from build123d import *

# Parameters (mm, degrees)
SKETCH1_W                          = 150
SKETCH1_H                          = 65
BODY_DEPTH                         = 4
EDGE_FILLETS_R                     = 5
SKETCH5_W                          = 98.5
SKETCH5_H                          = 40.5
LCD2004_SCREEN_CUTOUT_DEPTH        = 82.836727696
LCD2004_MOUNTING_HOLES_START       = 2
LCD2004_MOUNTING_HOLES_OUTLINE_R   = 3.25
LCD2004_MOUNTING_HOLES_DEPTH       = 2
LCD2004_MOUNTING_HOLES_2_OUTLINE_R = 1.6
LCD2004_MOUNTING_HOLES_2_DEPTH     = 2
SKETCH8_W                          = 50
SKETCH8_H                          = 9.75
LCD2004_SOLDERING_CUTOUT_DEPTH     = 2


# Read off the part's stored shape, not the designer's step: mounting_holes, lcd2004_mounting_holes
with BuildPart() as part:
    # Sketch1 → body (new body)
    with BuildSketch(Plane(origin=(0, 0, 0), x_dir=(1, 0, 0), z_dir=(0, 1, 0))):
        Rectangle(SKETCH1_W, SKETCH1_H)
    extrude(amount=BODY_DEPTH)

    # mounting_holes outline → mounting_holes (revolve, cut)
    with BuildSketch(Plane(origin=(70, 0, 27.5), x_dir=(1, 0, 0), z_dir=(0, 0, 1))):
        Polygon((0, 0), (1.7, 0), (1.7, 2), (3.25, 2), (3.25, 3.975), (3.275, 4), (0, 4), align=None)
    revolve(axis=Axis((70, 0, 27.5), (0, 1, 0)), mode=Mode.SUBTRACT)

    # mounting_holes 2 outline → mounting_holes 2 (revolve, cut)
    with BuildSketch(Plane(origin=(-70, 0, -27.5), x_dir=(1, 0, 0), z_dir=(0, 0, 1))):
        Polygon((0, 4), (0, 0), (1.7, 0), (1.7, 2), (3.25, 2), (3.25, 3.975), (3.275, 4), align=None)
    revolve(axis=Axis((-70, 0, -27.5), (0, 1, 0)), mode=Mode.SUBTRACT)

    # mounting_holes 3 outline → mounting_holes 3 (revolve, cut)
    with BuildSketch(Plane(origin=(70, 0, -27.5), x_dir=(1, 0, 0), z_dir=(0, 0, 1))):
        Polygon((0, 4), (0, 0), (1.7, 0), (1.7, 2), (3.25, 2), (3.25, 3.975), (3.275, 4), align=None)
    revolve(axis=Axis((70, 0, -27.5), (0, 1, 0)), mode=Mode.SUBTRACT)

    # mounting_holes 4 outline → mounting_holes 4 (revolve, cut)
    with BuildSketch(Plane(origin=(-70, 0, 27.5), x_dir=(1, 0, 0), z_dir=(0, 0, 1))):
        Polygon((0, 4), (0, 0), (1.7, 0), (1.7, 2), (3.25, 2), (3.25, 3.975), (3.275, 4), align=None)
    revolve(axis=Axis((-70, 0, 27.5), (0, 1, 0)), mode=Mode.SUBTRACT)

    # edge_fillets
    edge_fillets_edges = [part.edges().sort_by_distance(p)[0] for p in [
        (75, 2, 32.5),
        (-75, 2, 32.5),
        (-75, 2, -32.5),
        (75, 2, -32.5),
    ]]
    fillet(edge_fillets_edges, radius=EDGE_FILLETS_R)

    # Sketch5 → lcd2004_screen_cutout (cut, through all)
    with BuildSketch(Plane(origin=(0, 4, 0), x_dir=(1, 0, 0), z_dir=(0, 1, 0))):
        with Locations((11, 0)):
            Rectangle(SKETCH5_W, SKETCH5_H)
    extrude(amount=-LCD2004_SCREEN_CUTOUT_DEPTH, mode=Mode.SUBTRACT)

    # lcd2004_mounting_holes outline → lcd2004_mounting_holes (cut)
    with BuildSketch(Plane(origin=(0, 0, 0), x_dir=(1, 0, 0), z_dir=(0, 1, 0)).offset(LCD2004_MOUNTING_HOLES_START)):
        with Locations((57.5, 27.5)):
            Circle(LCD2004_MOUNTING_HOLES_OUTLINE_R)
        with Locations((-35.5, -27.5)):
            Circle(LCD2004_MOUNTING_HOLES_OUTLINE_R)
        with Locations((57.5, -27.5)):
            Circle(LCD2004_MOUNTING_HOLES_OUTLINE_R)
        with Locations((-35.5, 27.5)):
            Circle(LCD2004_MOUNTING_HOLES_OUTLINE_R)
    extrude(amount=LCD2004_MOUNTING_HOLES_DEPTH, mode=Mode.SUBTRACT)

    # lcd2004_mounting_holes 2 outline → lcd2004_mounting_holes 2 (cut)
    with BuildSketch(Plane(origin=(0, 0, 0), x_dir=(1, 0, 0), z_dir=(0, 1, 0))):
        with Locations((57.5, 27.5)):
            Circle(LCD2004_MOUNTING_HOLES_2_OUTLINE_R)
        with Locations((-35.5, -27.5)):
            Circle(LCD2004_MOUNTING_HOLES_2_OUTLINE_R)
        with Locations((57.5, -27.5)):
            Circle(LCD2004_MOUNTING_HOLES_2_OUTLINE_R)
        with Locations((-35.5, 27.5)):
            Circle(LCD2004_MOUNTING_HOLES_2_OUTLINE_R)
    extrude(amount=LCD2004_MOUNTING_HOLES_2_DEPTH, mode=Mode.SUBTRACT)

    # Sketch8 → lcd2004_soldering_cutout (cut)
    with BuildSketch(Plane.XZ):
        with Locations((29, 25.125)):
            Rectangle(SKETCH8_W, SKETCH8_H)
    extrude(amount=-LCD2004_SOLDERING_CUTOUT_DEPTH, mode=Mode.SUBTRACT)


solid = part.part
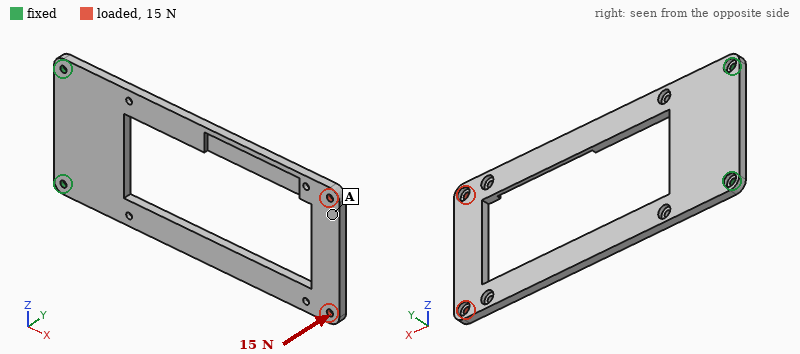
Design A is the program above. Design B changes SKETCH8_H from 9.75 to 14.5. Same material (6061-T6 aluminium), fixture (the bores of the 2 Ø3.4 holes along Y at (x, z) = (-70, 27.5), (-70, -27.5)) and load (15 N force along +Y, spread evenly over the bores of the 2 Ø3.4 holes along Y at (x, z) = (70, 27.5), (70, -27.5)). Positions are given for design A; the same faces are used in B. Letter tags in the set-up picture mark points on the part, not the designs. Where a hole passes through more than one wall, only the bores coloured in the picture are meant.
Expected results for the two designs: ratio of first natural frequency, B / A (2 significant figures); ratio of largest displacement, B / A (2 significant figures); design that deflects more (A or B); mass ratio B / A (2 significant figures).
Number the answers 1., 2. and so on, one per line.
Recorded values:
1. 0.97
2. 1.1
3. B
4. 0.99
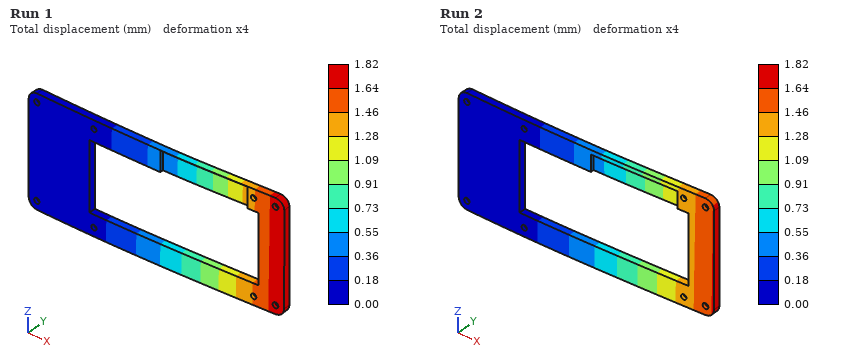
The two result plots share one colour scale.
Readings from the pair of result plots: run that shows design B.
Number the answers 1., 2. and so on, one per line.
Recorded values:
1. Run 1
